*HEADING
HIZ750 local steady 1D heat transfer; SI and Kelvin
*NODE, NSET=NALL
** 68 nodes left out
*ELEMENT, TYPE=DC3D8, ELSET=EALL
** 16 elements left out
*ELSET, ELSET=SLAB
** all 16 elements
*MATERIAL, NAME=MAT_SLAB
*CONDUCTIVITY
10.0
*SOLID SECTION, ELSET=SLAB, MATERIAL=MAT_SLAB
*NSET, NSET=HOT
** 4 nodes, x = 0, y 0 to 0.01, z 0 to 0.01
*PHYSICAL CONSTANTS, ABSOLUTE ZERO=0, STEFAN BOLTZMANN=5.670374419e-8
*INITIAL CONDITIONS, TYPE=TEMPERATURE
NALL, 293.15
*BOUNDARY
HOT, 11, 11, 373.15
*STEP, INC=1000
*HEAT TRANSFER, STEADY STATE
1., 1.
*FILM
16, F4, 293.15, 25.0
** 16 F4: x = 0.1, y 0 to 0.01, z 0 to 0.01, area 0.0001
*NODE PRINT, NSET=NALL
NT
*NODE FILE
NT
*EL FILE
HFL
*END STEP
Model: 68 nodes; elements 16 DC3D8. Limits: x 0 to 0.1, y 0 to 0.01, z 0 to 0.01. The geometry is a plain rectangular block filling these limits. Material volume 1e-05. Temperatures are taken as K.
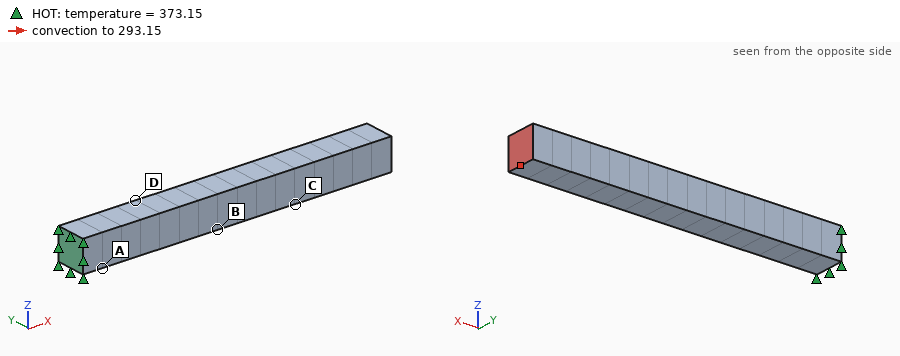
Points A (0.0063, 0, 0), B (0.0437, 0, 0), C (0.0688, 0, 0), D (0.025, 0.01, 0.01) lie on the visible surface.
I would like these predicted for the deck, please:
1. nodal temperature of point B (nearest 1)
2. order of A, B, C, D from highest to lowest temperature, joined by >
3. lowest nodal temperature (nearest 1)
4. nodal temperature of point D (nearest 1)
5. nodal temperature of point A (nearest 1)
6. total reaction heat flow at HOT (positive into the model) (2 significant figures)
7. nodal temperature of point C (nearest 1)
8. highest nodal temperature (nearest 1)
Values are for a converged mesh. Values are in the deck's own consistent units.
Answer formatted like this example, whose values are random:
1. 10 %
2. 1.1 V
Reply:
1. 366 K
2. A > D > B > C
3. 357 K
4. 369 K
5. 372 K
6. 0.16
7. 362 K
8. 373 K
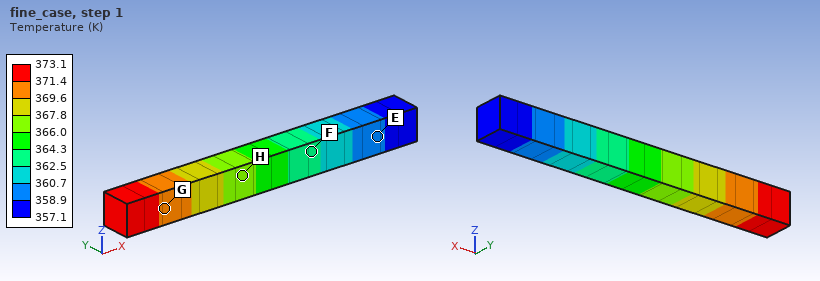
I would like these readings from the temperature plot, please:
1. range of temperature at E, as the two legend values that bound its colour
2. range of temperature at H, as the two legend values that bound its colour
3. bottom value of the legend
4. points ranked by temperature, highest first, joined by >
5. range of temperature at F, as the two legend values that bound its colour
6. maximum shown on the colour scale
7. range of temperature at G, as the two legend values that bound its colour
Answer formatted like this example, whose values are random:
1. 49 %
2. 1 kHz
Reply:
1. 358.9 to 360.7 K
2. 366.0 to 367.8 K
3. 357.1 K
4. G > H > F > E
5. 362.5 to 364.3 K
6. 373.1 K
7. 369.6 to 371.4 K
